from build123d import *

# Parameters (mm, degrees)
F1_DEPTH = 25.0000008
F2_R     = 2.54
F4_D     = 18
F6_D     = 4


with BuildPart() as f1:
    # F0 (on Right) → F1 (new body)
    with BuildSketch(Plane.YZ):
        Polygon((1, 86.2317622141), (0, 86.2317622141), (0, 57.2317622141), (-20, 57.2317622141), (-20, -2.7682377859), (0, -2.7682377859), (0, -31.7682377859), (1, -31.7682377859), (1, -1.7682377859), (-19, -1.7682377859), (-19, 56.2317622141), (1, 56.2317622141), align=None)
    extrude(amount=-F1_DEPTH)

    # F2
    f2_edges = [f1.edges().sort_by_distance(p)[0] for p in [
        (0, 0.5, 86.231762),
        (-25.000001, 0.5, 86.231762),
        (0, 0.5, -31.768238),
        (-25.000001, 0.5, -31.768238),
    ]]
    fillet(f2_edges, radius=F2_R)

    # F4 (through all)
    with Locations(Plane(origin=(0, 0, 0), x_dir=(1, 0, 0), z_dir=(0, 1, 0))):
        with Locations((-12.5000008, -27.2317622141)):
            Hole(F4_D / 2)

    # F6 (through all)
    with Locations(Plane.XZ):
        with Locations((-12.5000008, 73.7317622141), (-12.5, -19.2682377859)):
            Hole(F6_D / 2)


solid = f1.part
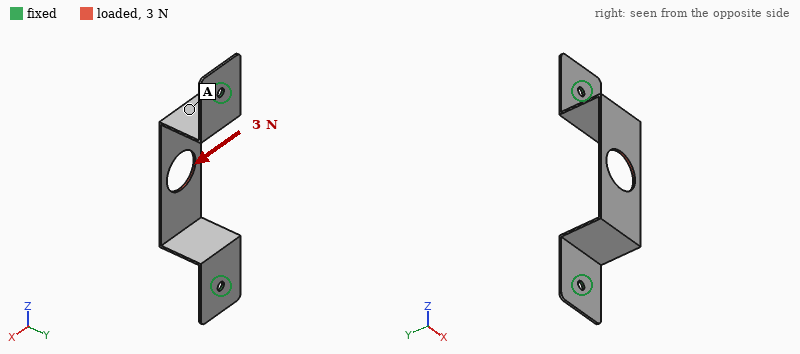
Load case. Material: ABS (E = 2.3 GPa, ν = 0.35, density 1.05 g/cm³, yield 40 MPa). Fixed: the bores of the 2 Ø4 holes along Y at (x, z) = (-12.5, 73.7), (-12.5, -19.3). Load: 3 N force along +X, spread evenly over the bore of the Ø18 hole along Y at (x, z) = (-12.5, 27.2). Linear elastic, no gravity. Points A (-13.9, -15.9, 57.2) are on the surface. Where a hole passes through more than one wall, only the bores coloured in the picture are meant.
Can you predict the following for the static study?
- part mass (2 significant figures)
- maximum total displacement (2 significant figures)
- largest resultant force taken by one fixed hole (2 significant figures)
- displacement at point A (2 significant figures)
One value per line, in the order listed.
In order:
3.8 g
1.2 mm
1.5 N
0.86 mm
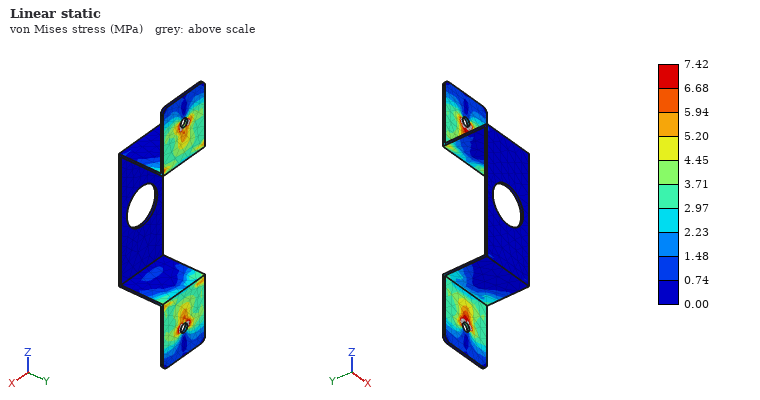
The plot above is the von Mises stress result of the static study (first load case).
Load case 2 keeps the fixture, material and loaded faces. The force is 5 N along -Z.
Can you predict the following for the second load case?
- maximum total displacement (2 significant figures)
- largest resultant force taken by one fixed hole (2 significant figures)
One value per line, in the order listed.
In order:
1.3 mm
2.7 N
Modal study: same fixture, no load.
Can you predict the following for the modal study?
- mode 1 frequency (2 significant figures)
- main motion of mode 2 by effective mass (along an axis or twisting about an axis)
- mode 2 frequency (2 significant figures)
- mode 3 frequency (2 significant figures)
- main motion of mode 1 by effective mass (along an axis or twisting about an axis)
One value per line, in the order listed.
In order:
190 Hz
along Z
230 Hz
300 Hz
along X
